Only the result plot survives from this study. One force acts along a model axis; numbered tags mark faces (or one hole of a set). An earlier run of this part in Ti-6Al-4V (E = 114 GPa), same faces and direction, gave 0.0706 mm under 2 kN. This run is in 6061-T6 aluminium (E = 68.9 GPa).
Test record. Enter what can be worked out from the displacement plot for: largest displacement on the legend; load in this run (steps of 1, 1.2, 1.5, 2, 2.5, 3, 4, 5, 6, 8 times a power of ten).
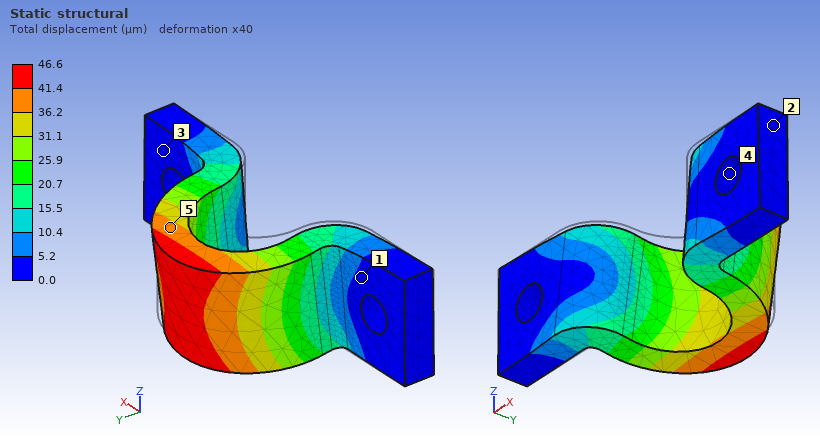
46.6 µm
800 N
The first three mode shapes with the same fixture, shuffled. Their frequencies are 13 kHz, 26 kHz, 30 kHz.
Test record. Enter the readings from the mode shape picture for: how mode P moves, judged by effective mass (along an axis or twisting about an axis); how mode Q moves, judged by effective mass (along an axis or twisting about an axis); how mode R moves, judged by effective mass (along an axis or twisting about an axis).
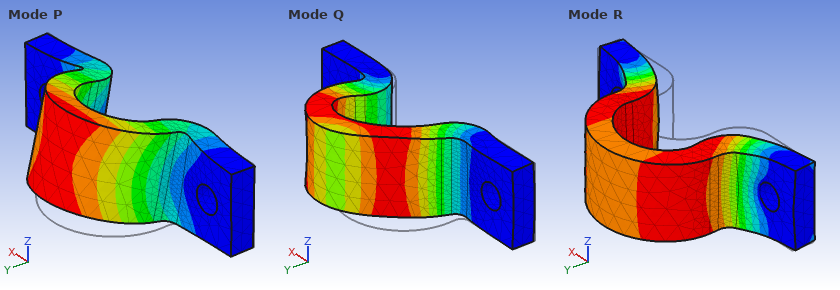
along Z
along X
along Y
